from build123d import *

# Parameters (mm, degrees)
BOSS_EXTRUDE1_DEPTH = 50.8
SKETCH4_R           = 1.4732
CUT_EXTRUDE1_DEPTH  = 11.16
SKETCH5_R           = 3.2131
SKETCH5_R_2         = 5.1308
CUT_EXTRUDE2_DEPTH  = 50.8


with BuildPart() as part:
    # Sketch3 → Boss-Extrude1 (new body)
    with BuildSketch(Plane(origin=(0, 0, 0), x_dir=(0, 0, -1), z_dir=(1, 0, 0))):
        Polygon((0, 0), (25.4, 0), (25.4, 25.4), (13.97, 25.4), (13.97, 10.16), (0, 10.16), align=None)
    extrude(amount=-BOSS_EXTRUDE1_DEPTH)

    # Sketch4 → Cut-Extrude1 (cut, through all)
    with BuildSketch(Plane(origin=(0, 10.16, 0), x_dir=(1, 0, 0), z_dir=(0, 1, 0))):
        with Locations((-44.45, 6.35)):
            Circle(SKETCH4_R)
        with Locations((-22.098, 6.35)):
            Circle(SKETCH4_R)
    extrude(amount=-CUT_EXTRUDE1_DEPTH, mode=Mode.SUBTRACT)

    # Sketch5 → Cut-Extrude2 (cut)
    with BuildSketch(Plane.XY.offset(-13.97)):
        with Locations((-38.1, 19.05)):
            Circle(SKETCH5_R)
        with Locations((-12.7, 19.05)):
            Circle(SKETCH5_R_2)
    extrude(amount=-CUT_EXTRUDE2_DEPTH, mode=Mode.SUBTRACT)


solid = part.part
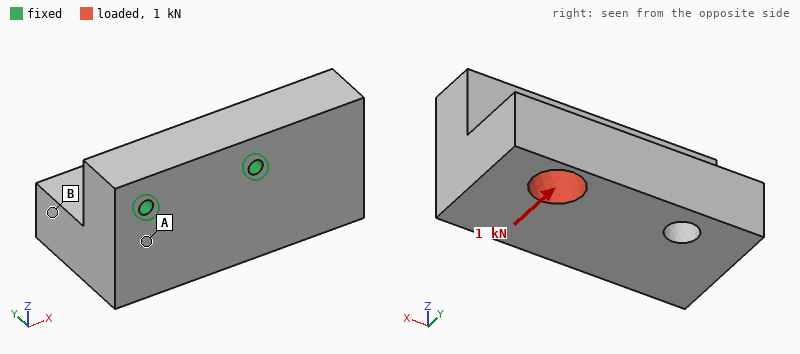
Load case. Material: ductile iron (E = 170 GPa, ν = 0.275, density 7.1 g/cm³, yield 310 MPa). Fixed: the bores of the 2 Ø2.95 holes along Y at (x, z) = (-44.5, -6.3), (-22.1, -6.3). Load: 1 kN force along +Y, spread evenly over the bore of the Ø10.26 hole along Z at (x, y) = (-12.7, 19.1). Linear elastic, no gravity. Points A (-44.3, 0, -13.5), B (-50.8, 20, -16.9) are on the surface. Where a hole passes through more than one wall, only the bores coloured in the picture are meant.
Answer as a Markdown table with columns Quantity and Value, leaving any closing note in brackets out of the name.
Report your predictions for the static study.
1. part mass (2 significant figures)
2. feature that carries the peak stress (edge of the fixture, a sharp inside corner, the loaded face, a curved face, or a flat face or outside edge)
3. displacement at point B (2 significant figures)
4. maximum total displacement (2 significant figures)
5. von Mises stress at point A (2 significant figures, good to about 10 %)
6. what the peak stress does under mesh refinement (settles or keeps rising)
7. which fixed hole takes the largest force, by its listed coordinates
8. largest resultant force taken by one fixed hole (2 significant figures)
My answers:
| Quantity | Value |
|---|---|
| part mass | 150 g |
| feature that carries the peak stress | edge of the fixture |
| displacement at point B | 3.1 µm |
| maximum total displacement | 13 µm |
| von Mises stress at point A | 13 MPa |
| what the peak stress does under mesh refinement | keeps rising |
| which fixed hole takes the largest force, by its listed coordinates | (-22.1, -6.3) |
| largest resultant force taken by one fixed hole | 1.2 kN |
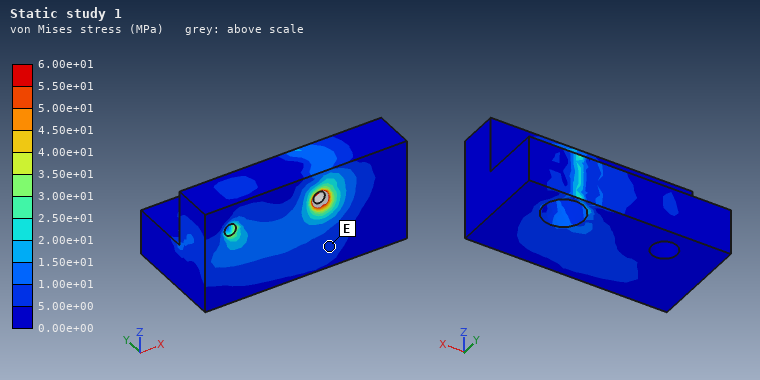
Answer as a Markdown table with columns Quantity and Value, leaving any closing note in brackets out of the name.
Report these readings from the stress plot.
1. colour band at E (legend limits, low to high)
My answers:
| Quantity | Value |
|---|---|
| colour band at E | 5.00e+00 to 1.00e+01 MPa |
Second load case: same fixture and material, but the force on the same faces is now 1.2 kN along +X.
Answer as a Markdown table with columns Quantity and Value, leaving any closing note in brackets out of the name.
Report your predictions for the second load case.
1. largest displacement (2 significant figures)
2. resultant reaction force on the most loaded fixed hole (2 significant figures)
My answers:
| Quantity | Value |
|---|---|
| largest displacement | 7.5 µm |
| resultant reaction force on the most loaded fixed hole | 1.1 kN |
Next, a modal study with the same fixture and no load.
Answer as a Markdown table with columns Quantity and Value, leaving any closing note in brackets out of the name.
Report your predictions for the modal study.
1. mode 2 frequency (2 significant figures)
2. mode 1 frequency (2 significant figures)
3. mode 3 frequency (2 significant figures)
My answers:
| Quantity | Value |
|---|---|
| mode 2 frequency | 9500 Hz |
| mode 1 frequency | 6600 Hz |
| mode 3 frequency | 12 kHz |
